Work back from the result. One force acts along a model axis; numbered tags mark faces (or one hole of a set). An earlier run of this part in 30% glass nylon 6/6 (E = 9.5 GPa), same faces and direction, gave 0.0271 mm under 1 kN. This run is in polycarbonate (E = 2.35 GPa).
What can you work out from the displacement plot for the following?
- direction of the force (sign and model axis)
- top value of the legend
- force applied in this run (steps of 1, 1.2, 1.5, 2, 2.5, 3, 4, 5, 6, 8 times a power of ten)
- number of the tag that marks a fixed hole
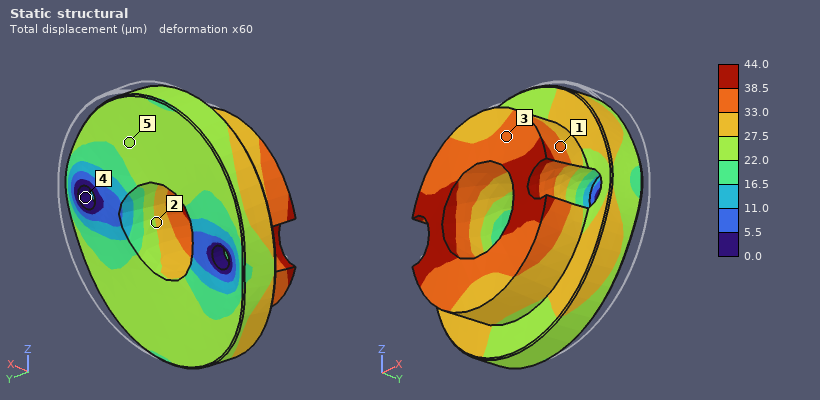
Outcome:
-X
44.0 µm
400 N
4
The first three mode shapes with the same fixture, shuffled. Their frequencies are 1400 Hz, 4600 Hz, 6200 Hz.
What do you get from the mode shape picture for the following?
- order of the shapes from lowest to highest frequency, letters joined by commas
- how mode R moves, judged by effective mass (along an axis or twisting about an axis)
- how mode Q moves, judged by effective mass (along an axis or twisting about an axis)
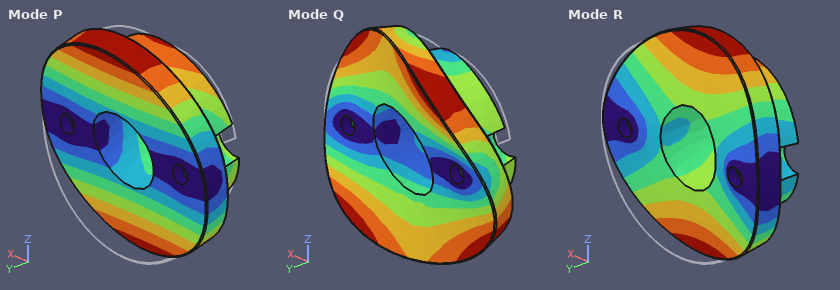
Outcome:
P, R, Q
along Y
twisting about Y
